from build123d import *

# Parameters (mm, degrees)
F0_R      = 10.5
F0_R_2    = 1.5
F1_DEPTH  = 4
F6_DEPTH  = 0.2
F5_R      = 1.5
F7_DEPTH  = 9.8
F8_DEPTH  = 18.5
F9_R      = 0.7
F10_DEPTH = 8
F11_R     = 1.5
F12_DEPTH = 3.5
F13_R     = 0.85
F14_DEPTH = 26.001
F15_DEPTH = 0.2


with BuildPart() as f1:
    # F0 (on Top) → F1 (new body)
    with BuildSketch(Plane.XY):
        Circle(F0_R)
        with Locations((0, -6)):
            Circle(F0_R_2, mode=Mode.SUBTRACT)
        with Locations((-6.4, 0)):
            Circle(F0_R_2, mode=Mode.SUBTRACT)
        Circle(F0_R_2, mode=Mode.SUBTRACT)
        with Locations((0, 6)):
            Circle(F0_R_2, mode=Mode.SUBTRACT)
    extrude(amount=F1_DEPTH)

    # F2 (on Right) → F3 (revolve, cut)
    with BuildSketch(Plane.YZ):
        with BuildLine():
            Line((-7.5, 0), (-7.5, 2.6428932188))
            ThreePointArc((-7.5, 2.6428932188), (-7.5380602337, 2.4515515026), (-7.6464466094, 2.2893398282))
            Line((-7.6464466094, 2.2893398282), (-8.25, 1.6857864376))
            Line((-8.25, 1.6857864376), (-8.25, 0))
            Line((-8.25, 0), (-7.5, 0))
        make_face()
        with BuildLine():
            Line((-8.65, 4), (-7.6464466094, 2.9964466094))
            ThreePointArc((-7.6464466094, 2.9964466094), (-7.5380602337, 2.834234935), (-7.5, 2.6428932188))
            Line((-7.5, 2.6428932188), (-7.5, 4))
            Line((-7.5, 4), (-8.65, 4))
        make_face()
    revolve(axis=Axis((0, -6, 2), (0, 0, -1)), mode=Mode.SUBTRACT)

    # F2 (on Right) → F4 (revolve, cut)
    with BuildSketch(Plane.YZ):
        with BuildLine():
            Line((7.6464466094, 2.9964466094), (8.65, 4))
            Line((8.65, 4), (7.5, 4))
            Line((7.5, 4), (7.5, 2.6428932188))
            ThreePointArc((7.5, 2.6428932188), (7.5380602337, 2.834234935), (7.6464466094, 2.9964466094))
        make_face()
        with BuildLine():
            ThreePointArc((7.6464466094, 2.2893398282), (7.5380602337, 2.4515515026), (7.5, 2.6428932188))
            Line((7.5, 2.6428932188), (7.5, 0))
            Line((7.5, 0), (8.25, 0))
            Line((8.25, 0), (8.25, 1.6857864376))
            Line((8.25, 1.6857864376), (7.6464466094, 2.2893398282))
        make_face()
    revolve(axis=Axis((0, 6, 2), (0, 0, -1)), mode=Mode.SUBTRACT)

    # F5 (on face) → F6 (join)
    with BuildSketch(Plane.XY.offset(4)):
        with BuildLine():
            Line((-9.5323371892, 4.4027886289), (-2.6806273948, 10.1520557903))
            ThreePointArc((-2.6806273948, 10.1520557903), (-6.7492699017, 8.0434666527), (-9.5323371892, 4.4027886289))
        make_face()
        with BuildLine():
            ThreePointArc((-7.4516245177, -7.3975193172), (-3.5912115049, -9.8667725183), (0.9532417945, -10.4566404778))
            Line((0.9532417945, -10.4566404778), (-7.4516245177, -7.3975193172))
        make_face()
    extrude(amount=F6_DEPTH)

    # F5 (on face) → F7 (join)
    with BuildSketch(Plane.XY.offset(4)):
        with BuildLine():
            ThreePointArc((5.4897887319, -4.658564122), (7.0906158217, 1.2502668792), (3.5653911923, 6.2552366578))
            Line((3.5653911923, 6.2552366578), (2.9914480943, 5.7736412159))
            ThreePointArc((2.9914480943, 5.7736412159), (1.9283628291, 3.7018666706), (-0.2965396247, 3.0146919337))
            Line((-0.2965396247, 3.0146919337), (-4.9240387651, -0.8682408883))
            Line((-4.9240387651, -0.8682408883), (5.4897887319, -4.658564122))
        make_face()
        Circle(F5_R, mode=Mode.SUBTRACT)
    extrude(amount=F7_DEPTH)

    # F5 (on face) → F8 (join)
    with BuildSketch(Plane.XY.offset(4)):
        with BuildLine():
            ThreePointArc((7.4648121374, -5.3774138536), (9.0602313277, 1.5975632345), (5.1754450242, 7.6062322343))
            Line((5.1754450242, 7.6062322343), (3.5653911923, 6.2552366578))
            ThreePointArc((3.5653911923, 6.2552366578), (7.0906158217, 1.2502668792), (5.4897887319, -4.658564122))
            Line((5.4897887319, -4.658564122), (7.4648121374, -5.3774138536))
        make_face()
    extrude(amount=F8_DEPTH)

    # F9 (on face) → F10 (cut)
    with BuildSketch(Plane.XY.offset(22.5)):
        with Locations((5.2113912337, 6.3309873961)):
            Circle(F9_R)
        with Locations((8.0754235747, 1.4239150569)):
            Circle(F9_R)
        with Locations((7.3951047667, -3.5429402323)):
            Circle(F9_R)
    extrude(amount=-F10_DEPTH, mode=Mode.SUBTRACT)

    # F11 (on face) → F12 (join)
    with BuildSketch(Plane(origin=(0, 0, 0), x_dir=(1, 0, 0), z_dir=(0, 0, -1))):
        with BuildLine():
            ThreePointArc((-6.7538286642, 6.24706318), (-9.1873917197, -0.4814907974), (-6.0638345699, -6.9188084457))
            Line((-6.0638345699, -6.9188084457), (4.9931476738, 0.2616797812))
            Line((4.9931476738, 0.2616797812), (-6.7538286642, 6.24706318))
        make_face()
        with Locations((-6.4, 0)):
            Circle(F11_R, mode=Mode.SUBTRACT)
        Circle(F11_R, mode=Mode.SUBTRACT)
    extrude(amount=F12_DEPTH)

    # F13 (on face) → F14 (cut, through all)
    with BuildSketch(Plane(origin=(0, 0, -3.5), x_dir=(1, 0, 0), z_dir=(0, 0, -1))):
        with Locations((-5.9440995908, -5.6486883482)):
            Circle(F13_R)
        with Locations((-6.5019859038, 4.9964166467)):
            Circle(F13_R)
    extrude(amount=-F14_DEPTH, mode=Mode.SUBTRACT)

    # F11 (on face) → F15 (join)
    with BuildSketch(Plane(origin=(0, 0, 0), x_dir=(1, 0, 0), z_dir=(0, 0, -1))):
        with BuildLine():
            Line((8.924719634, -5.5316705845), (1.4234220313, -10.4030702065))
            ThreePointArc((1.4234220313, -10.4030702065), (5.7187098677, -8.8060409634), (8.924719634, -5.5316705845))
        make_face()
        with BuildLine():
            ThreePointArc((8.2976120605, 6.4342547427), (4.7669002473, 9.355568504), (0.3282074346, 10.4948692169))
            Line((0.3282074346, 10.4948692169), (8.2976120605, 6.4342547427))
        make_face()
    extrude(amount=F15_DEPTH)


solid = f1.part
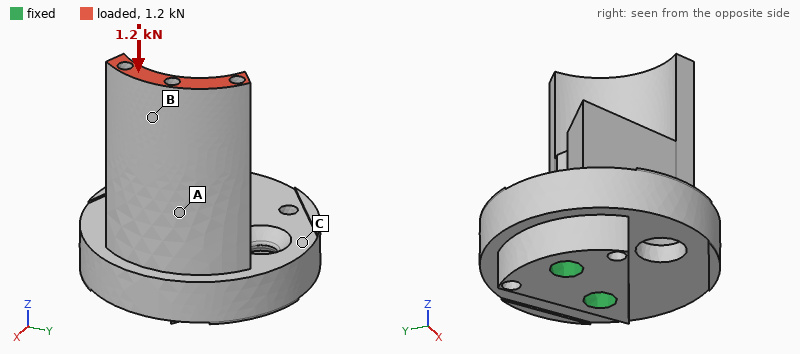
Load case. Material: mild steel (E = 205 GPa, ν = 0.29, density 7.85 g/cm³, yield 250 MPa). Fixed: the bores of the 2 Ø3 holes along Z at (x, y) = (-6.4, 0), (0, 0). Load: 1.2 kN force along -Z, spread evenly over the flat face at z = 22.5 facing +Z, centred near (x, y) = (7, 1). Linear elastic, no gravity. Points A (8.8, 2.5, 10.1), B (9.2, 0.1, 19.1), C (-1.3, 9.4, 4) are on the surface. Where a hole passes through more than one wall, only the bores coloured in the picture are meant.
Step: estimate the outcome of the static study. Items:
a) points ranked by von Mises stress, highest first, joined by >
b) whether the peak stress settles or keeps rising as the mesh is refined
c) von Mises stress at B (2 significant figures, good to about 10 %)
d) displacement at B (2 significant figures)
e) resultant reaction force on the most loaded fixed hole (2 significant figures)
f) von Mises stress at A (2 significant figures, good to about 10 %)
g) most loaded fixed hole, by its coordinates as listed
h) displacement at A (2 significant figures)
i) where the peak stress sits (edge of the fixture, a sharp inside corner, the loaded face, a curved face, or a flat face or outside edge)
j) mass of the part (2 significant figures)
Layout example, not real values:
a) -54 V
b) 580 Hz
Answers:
a) B > A > C
b) keeps rising
c) 53 MPa
d) 4.8 µm
e) 1.2 kN
f) 38 MPa
g) (0, 0)
h) 1.7 µm
i) edge of the fixture
j) 20 g
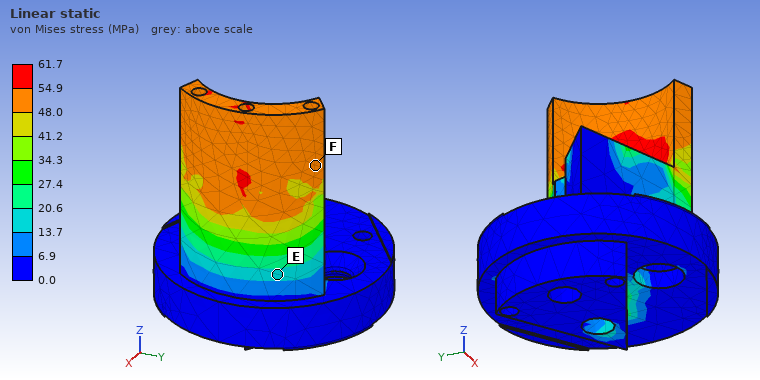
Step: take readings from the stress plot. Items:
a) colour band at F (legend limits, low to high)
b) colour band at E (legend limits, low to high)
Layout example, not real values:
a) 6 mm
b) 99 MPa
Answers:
a) 48.0 to 54.9 MPa
b) 13.7 to 20.6 MPa
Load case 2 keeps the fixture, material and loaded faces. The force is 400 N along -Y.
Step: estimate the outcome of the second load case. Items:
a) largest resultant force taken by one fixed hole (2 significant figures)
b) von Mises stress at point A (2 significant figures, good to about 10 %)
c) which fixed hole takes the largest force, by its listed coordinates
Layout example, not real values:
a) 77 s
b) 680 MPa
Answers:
a) 470 N
b) 25 MPa
c) (0, 0)
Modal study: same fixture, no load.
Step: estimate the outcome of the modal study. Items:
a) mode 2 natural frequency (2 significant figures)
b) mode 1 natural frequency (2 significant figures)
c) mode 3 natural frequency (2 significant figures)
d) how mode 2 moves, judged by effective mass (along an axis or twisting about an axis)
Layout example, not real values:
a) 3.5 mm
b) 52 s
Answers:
a) 28 kHz
b) 22 kHz
c) 32 kHz
d) along Y
